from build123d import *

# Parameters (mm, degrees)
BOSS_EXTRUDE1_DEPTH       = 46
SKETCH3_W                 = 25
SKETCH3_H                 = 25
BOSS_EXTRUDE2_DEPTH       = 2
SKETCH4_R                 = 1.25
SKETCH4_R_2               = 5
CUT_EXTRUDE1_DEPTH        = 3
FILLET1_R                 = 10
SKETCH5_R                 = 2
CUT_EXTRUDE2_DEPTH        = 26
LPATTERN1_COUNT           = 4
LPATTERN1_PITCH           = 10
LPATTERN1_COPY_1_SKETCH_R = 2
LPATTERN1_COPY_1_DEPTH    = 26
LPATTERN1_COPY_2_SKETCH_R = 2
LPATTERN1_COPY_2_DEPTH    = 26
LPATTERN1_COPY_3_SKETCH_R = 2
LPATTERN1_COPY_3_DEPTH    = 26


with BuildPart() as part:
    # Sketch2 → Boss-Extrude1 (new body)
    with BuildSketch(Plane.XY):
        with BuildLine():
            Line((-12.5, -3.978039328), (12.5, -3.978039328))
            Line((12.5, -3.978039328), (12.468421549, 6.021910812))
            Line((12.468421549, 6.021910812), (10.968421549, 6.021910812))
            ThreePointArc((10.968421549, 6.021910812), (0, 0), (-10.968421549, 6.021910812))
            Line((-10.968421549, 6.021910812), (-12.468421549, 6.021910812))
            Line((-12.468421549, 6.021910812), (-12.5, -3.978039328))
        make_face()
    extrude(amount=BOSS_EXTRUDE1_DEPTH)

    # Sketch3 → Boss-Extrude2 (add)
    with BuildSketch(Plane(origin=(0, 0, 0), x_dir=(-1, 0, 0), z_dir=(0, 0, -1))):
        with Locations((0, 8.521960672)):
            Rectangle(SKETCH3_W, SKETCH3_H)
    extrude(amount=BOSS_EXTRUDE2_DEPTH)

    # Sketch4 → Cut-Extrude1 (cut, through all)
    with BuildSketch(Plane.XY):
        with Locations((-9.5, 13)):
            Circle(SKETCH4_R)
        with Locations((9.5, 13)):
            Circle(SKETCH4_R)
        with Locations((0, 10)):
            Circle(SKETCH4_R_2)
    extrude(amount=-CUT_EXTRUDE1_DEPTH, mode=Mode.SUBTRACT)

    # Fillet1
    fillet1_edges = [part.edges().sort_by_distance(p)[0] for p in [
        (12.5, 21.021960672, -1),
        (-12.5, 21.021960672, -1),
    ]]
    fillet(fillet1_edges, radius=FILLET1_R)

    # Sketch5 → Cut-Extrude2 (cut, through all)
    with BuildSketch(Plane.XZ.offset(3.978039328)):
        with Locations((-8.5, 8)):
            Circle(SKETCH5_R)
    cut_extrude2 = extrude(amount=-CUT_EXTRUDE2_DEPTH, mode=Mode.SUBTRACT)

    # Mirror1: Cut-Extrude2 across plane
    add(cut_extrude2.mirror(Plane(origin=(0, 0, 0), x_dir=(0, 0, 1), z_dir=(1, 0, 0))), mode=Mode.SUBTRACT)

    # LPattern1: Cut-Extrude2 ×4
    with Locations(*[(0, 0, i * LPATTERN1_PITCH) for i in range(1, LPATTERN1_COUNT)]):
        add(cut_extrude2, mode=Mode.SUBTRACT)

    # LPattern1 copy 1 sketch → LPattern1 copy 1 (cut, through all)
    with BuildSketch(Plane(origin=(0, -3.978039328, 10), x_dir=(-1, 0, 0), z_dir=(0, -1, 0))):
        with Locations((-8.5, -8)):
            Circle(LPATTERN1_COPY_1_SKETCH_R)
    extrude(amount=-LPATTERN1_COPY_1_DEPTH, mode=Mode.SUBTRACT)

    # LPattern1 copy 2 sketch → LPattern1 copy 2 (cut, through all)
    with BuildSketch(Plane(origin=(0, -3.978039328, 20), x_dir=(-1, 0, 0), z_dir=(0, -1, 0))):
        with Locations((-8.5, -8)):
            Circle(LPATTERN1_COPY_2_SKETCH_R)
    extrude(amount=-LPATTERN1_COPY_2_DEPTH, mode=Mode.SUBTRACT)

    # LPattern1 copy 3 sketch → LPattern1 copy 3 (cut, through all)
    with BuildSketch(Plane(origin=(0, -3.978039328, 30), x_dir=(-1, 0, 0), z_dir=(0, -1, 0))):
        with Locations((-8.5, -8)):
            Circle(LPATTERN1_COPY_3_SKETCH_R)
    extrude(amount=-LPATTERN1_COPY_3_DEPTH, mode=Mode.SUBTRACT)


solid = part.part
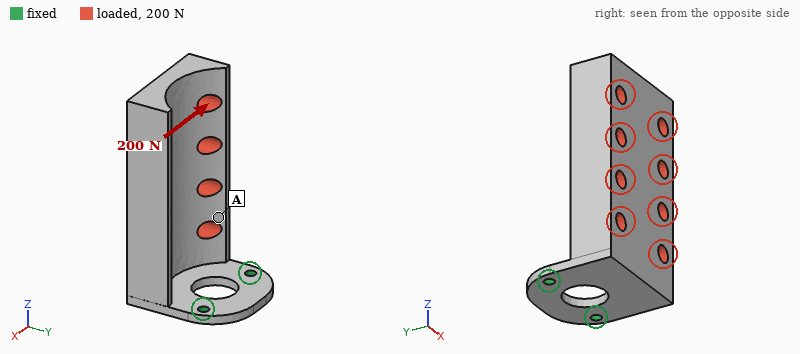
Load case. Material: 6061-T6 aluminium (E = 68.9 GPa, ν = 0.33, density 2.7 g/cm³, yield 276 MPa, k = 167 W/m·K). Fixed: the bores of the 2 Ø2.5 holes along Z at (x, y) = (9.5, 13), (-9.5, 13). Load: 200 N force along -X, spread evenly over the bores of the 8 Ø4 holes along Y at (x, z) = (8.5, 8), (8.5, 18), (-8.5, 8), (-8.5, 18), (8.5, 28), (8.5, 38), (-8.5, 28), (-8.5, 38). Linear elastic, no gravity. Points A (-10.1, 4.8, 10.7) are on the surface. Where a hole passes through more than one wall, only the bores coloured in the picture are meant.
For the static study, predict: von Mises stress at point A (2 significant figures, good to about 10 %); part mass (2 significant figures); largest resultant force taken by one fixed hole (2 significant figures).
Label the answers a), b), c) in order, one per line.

a) 20 MPa
b) 20 g
c) 270 N
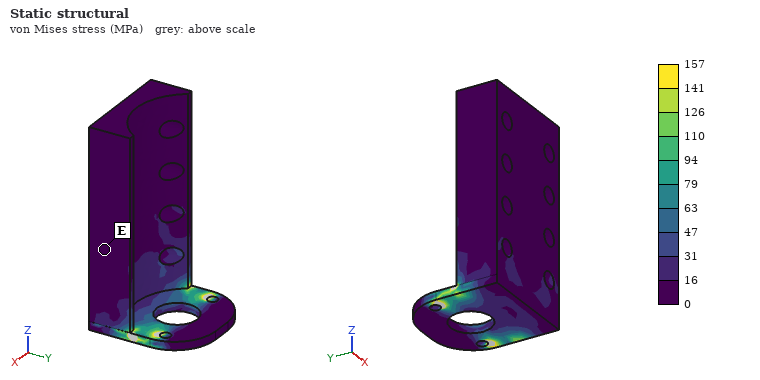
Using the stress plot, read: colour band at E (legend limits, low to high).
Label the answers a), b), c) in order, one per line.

a) 0 to 16 MPa
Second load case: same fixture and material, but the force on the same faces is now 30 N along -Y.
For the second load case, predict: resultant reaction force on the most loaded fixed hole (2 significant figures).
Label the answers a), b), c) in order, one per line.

a) 16 N
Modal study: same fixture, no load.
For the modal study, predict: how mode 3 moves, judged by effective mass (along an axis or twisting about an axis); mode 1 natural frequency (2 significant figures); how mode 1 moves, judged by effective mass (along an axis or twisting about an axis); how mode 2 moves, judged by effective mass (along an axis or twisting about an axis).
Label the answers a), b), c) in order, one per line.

a) along Z
b) 390 Hz
c) along Y
d) along X
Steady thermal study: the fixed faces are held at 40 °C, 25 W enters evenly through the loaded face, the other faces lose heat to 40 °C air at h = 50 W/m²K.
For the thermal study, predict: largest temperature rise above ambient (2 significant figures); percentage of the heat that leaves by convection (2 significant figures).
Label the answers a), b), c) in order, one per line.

a) 50 K
b) 33 %
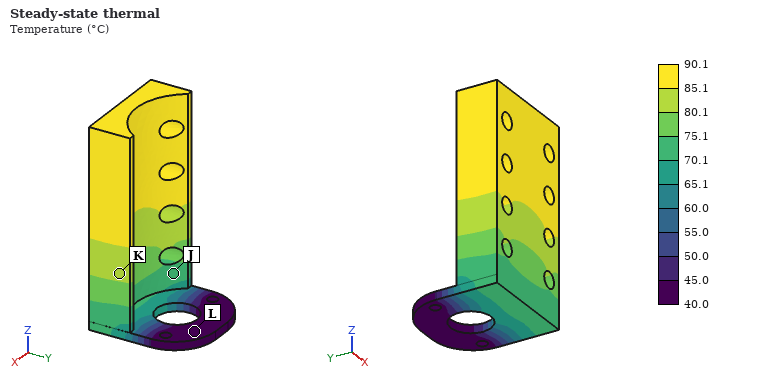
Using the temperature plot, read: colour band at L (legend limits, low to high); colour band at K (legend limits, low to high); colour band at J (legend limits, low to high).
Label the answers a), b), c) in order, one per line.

a) 40.0 to 45.0 °C
b) 80.1 to 85.1 °C
c) 70.1 to 75.1 °C
